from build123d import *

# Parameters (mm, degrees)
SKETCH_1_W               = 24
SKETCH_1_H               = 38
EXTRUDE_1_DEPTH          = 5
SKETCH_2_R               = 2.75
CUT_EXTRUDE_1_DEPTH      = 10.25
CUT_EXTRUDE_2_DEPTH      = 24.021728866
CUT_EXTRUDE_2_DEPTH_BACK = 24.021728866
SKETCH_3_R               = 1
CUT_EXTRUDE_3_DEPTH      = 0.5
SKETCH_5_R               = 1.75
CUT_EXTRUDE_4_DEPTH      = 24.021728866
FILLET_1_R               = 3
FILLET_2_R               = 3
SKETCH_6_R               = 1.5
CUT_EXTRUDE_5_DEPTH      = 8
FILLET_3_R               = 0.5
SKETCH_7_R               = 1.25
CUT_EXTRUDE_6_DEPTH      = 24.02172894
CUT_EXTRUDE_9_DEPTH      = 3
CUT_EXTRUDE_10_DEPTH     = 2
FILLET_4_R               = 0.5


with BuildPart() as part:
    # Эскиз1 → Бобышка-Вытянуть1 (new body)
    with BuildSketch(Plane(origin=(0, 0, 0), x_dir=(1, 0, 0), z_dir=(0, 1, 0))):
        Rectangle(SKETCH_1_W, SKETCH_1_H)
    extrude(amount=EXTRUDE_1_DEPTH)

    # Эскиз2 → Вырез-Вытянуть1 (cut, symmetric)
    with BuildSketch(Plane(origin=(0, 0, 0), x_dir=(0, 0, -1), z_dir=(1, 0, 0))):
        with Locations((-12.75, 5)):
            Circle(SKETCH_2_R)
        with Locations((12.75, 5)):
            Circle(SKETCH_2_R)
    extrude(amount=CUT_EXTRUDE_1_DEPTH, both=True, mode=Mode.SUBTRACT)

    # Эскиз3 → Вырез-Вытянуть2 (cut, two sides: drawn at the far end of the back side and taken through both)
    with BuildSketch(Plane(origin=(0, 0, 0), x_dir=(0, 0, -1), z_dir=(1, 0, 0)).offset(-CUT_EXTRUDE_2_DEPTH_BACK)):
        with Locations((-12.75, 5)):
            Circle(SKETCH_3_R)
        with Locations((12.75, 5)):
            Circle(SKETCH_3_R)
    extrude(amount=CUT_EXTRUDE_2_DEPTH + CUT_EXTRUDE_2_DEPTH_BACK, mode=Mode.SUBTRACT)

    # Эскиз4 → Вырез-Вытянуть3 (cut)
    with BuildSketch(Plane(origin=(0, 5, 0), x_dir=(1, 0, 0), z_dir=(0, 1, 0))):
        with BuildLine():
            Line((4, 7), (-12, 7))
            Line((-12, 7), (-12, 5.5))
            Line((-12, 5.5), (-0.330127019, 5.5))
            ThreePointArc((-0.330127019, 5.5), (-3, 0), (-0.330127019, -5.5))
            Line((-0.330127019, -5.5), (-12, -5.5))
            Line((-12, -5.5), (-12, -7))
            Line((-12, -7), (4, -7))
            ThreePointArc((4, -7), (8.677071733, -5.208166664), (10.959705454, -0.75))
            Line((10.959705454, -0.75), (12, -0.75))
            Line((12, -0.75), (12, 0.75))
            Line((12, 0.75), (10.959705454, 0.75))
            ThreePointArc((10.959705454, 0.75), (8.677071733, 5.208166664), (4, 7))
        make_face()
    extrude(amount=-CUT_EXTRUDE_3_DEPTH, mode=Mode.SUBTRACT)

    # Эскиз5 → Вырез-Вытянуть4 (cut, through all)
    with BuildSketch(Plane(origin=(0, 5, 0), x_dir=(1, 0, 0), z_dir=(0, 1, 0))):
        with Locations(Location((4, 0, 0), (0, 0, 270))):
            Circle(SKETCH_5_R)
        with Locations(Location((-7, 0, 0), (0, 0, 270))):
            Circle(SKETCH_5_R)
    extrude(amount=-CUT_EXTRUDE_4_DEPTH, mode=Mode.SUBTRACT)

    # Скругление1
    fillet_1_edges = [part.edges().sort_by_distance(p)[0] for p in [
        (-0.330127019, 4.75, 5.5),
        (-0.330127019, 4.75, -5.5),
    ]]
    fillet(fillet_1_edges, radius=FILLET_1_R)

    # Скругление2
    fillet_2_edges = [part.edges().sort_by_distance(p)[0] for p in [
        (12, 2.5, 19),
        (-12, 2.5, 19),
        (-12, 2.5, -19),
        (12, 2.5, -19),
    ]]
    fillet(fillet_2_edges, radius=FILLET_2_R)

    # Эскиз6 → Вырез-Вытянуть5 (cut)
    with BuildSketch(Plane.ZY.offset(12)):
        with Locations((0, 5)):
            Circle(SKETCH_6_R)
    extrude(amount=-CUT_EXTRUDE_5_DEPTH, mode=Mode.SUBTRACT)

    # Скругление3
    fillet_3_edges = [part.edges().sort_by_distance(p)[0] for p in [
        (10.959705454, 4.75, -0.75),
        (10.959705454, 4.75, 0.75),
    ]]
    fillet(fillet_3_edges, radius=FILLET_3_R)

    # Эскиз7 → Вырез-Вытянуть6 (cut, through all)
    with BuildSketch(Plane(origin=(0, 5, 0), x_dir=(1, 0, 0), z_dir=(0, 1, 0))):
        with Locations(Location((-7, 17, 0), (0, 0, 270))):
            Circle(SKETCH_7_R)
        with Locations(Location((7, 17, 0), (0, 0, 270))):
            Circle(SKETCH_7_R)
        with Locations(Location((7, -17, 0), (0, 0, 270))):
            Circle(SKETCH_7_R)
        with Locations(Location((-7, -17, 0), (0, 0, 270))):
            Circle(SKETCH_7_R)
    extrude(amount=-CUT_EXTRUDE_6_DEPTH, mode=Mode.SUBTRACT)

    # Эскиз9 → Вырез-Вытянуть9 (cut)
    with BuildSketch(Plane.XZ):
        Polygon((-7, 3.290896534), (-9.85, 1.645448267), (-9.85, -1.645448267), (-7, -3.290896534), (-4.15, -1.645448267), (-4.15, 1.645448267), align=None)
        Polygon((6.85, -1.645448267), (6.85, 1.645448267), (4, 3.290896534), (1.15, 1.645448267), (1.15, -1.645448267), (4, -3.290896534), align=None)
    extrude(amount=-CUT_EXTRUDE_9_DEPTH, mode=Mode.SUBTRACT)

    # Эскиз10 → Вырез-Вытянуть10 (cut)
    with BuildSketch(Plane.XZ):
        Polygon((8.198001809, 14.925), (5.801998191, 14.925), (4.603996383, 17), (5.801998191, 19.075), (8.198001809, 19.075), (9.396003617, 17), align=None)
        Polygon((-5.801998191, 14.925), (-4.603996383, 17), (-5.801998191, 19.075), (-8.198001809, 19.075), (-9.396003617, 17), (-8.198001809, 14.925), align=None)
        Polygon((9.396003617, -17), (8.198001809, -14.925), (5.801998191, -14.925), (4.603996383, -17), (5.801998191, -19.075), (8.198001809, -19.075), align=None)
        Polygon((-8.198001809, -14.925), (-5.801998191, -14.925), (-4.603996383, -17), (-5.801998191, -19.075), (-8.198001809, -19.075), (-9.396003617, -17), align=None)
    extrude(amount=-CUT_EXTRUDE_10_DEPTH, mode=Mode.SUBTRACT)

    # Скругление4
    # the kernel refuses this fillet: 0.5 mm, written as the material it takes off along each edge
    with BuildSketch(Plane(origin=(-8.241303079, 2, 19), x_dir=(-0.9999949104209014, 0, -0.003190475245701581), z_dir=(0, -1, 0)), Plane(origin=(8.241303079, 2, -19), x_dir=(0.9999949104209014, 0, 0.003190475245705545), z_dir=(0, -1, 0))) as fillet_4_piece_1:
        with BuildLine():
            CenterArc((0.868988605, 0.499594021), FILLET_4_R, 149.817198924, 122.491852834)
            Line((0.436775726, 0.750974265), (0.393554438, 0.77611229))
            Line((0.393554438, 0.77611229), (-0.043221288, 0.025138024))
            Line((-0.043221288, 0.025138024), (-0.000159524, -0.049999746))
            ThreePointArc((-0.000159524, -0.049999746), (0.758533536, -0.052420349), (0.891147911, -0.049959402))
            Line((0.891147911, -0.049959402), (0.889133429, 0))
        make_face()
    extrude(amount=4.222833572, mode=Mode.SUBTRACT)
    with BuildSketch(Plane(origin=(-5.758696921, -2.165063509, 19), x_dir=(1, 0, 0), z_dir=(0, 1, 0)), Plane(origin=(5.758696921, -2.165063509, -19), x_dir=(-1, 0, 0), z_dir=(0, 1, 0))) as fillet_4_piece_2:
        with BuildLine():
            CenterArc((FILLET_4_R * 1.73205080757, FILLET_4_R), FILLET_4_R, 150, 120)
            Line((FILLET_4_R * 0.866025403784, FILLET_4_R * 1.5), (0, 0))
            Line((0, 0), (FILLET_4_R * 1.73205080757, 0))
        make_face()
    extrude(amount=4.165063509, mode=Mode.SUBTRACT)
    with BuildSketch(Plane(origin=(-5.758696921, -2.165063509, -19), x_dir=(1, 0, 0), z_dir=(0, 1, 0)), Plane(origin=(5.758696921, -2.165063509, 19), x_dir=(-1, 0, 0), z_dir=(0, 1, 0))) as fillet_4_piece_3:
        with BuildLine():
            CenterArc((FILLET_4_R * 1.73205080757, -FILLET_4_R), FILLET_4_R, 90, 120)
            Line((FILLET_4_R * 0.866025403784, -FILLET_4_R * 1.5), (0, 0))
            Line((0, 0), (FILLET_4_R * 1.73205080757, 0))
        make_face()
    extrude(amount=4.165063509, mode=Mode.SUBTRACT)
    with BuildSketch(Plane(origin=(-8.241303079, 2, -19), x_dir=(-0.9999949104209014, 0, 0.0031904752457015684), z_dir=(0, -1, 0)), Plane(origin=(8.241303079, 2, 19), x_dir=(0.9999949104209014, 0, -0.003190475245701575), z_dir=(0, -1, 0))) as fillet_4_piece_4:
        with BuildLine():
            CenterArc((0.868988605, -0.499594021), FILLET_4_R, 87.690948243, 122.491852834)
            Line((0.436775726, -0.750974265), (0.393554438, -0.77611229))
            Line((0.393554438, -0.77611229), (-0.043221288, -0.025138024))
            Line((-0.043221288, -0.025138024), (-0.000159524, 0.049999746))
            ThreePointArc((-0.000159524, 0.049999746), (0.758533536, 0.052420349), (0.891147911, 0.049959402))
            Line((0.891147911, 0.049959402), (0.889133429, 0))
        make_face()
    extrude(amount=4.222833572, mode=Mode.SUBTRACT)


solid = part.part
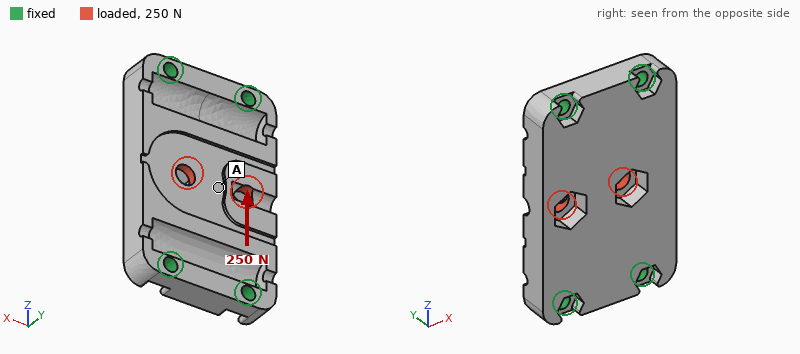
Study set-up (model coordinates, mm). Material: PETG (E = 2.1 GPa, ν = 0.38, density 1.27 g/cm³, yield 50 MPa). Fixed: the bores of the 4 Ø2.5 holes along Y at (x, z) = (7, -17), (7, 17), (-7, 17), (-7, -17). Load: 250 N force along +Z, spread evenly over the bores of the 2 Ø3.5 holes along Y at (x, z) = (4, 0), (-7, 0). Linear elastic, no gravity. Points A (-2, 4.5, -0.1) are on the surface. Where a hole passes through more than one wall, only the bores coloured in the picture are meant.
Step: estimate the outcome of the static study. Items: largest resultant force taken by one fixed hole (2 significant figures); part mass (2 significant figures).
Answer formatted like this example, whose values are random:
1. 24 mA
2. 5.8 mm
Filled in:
1. 65 N
2. 4.5 g
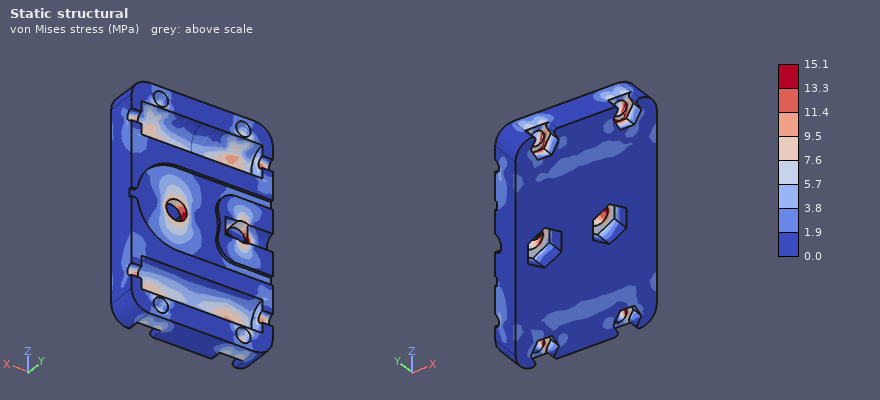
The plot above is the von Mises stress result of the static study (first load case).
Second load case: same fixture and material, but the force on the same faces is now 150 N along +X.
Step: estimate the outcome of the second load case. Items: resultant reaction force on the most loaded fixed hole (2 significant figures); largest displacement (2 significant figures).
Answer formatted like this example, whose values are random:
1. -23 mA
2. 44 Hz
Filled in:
1. 41 N
2. 77 µm
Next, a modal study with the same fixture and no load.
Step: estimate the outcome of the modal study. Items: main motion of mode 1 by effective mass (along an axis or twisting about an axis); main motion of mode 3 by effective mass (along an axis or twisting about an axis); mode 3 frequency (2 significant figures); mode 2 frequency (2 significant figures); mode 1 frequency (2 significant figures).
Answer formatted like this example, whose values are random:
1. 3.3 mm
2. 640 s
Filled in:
1. along Y
2. along Z
3. 7200 Hz
4. 4100 Hz
5. 3000 Hz
